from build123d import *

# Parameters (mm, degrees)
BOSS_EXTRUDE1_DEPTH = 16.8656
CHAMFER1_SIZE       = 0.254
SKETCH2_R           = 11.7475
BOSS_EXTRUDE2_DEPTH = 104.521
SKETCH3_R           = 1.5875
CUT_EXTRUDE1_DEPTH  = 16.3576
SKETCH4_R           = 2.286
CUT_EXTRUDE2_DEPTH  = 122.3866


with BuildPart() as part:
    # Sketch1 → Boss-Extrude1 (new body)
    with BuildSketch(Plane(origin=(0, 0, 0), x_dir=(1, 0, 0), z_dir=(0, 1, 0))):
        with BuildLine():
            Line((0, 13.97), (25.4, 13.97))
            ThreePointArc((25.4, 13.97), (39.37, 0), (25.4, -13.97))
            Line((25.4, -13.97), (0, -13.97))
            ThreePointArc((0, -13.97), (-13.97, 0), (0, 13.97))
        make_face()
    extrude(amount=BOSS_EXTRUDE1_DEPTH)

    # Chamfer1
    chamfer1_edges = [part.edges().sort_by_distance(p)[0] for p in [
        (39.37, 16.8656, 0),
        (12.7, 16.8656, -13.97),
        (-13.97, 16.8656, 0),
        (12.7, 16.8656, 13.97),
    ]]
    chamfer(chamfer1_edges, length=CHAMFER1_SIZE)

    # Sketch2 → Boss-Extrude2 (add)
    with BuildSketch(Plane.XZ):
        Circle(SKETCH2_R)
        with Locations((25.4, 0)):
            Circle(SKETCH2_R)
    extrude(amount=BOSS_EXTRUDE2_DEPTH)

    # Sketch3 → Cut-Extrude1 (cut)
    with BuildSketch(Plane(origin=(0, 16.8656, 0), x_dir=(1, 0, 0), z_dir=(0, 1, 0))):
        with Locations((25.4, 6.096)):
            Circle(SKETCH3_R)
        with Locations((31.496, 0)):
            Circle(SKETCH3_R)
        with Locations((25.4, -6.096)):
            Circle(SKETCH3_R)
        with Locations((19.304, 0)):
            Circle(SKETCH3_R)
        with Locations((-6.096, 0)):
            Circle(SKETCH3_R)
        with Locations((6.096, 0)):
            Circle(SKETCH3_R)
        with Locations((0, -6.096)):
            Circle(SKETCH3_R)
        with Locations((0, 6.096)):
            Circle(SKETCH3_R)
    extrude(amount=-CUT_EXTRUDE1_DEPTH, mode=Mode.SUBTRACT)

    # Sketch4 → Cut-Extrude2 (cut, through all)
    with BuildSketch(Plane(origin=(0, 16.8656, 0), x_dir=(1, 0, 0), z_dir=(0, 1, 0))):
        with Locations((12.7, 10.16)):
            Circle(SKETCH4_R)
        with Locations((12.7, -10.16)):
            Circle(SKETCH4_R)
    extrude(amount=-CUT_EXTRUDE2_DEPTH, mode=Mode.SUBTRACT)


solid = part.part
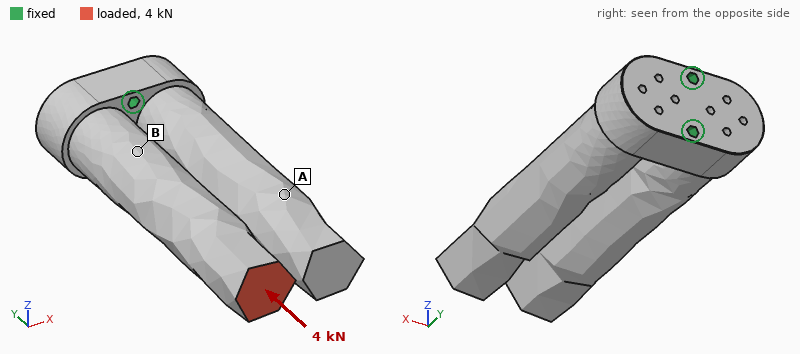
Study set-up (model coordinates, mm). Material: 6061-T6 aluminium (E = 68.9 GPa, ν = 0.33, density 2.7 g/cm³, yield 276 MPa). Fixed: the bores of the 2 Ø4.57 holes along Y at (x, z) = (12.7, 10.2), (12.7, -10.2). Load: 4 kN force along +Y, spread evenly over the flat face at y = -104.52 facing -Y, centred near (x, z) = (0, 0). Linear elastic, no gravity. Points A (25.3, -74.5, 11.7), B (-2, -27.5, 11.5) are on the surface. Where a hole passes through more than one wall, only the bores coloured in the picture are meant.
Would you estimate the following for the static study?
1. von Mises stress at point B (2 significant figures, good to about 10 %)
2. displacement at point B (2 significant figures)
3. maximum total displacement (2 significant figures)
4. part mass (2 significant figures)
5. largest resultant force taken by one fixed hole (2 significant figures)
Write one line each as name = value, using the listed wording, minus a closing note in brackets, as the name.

von Mises stress at point B = 9.1 MPa
displacement at point B = 26 µm
maximum total displacement = 77 µm
part mass = 300 g
largest resultant force taken by one fixed hole = 2.0 kN
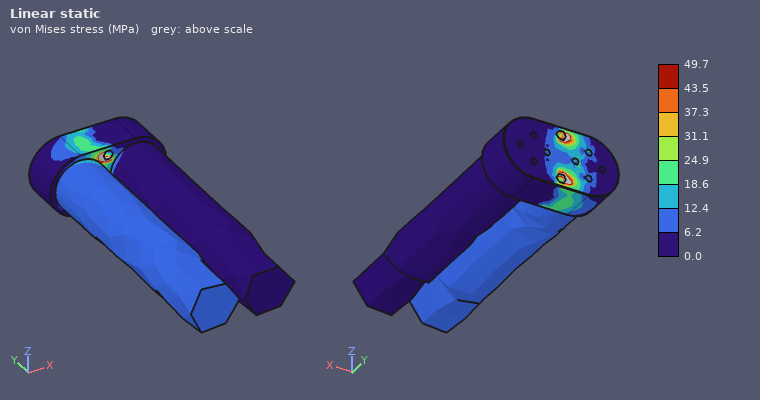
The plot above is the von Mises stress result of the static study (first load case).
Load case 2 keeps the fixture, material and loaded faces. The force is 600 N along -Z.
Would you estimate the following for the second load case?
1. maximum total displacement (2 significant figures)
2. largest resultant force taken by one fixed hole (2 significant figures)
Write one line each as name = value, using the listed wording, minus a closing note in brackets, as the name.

maximum total displacement = 0.31 mm
largest resultant force taken by one fixed hole = 2.7 kN
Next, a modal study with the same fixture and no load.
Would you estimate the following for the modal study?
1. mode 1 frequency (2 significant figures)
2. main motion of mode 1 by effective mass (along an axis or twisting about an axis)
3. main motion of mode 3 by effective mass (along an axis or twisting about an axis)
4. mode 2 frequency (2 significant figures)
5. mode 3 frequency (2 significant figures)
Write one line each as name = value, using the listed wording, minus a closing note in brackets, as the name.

mode 1 frequency = 1100 Hz
main motion of mode 1 by effective mass = along X
main motion of mode 3 by effective mass = along Z
mode 2 frequency = 1100 Hz
mode 3 frequency = 1200 Hz
